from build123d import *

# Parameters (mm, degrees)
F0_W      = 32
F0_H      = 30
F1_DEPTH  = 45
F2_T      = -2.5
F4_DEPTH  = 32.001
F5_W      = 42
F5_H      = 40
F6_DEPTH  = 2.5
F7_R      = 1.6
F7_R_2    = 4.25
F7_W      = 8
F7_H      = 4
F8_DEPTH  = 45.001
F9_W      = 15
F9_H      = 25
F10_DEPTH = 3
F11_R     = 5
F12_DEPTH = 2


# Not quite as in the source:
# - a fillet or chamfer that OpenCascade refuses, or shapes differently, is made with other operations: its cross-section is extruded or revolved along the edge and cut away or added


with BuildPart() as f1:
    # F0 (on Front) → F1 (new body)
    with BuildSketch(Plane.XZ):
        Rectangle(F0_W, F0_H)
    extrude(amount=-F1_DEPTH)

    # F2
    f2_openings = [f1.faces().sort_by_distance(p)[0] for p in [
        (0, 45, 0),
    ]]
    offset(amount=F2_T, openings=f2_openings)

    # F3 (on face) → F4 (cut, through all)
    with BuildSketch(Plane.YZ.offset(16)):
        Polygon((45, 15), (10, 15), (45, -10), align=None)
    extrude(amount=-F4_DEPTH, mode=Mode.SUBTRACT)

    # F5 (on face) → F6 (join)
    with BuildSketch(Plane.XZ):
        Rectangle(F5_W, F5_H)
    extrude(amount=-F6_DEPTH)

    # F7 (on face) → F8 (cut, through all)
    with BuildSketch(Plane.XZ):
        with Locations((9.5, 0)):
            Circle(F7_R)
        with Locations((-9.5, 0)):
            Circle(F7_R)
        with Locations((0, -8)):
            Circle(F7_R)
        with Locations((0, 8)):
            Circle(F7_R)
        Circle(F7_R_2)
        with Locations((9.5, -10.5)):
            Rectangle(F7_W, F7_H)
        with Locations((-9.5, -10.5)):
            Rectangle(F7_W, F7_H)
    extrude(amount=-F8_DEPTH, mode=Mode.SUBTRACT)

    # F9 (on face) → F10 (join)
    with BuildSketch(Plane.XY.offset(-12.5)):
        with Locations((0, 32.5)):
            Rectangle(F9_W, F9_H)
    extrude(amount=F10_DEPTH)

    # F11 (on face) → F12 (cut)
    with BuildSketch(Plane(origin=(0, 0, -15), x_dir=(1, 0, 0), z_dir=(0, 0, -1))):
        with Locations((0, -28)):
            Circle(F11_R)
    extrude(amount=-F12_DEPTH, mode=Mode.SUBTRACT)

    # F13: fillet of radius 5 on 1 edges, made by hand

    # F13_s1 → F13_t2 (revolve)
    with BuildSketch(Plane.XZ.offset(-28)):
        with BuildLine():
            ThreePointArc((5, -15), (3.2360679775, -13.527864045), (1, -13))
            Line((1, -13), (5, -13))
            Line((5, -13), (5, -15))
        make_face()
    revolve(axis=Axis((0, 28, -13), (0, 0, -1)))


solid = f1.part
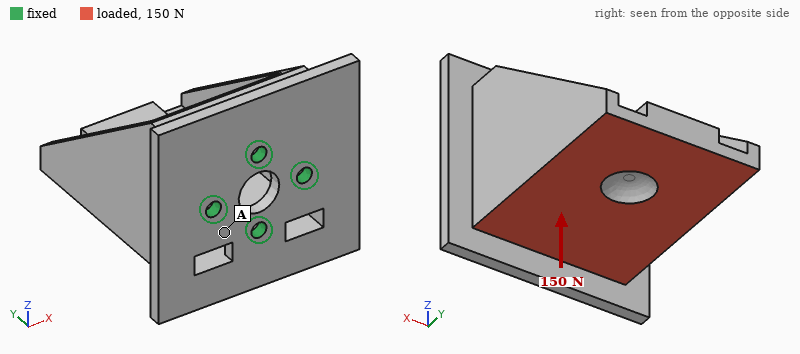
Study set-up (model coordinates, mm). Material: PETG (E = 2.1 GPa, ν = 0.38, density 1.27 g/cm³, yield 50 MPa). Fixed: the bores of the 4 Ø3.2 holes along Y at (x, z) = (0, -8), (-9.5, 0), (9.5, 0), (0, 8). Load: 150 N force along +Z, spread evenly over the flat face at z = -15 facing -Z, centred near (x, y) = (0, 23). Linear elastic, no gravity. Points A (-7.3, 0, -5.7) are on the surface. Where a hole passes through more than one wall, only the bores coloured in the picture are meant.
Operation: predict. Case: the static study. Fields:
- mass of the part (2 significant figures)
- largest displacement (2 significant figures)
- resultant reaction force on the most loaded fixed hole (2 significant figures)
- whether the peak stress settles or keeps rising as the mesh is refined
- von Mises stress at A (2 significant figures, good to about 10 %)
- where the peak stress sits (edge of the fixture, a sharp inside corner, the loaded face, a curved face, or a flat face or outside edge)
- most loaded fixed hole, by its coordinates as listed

16 g
0.80 mm
130 N
keeps rising
4.2 MPa
edge of the fixture
(0, -8)
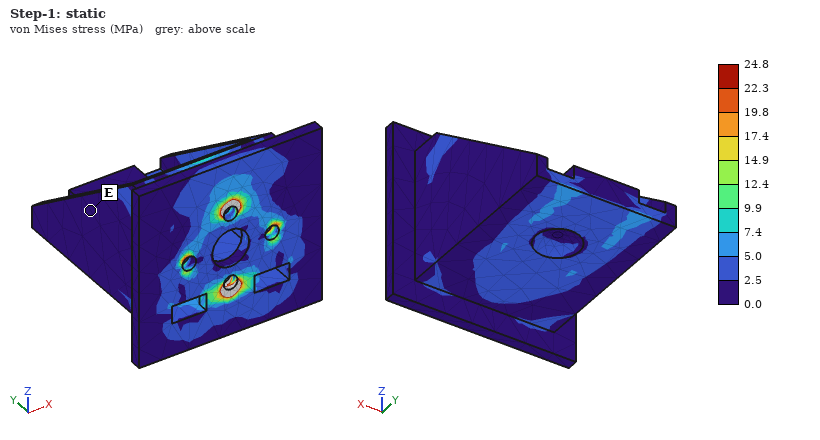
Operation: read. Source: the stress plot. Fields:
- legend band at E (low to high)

0.0 to 2.5 MPa
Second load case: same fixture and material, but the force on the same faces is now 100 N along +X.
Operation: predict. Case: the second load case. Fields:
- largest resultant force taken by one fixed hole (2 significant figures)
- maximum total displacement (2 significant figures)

89 N
0.76 mm
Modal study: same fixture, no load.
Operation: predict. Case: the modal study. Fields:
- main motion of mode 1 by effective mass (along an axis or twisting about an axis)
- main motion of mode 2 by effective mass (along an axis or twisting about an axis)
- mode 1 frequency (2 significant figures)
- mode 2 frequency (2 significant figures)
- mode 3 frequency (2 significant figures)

along X
along Z
660 Hz
840 Hz
1600 Hz
